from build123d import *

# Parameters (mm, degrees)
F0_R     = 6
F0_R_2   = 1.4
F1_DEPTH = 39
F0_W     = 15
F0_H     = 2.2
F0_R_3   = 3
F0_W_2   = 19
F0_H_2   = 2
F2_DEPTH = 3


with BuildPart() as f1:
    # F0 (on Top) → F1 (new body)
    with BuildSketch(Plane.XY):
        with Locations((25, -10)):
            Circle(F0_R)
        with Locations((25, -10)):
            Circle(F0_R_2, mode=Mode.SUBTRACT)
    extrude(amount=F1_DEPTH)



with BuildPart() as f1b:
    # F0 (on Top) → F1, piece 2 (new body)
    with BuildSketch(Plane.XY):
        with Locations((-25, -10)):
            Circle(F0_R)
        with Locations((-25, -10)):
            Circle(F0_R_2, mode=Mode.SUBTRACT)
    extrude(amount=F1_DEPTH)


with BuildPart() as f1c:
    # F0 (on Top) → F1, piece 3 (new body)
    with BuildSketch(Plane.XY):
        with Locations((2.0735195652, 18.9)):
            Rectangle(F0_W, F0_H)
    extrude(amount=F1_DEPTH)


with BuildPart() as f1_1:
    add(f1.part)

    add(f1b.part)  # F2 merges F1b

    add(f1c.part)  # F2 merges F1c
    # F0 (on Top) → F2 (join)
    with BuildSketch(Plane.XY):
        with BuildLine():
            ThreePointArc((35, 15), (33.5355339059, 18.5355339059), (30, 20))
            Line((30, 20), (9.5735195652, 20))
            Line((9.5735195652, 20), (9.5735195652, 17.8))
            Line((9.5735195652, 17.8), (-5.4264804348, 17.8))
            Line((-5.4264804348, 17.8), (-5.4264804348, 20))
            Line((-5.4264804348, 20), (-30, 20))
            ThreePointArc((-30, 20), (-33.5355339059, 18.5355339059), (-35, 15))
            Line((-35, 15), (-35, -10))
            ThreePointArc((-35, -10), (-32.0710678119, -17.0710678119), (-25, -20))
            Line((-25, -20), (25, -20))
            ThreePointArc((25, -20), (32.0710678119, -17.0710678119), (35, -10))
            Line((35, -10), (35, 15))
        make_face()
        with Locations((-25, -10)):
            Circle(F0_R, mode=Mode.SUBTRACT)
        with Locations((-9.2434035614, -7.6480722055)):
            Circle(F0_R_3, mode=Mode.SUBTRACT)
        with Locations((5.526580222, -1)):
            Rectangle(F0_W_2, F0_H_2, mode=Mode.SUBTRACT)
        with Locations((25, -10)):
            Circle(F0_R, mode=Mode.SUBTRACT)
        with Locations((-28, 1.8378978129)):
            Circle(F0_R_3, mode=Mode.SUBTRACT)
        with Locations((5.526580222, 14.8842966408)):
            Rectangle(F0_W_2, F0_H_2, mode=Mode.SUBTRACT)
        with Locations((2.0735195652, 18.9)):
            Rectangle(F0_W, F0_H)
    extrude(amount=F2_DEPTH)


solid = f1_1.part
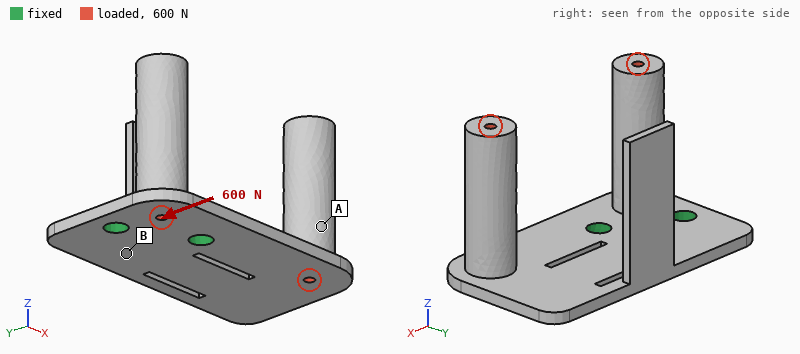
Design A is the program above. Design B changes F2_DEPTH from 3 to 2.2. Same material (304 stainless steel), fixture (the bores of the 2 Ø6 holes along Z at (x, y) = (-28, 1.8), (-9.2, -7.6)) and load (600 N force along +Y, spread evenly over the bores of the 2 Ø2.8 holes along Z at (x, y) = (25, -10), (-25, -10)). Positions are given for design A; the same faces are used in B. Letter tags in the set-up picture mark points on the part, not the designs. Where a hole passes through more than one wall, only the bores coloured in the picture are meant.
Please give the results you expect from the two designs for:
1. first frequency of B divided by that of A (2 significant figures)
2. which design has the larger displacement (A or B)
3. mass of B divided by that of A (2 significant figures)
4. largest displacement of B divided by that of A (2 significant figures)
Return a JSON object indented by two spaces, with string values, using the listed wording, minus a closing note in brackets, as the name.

{
  "first frequency of B divided by that of A": "0.65",
  "which design has the larger displacement": "B",
  "mass of B divided by that of A": "0.89",
  "largest displacement of B divided by that of A": "2.4"
}
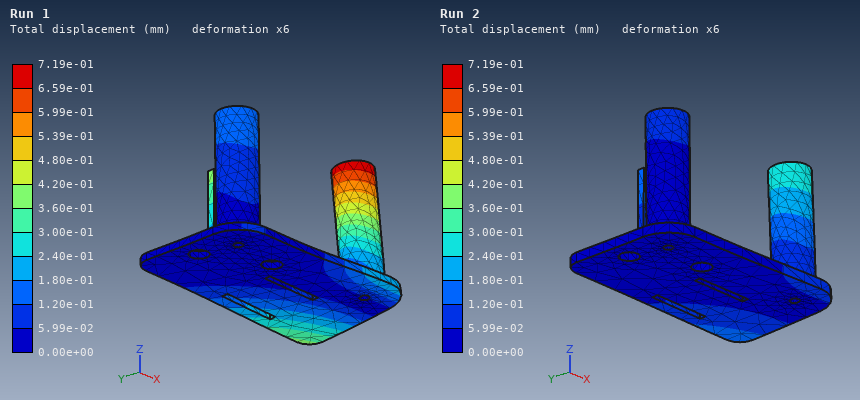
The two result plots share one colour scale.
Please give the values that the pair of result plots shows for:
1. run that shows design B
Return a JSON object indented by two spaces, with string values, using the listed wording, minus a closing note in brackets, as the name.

{
  "run that shows design B": "Run 1"
}
